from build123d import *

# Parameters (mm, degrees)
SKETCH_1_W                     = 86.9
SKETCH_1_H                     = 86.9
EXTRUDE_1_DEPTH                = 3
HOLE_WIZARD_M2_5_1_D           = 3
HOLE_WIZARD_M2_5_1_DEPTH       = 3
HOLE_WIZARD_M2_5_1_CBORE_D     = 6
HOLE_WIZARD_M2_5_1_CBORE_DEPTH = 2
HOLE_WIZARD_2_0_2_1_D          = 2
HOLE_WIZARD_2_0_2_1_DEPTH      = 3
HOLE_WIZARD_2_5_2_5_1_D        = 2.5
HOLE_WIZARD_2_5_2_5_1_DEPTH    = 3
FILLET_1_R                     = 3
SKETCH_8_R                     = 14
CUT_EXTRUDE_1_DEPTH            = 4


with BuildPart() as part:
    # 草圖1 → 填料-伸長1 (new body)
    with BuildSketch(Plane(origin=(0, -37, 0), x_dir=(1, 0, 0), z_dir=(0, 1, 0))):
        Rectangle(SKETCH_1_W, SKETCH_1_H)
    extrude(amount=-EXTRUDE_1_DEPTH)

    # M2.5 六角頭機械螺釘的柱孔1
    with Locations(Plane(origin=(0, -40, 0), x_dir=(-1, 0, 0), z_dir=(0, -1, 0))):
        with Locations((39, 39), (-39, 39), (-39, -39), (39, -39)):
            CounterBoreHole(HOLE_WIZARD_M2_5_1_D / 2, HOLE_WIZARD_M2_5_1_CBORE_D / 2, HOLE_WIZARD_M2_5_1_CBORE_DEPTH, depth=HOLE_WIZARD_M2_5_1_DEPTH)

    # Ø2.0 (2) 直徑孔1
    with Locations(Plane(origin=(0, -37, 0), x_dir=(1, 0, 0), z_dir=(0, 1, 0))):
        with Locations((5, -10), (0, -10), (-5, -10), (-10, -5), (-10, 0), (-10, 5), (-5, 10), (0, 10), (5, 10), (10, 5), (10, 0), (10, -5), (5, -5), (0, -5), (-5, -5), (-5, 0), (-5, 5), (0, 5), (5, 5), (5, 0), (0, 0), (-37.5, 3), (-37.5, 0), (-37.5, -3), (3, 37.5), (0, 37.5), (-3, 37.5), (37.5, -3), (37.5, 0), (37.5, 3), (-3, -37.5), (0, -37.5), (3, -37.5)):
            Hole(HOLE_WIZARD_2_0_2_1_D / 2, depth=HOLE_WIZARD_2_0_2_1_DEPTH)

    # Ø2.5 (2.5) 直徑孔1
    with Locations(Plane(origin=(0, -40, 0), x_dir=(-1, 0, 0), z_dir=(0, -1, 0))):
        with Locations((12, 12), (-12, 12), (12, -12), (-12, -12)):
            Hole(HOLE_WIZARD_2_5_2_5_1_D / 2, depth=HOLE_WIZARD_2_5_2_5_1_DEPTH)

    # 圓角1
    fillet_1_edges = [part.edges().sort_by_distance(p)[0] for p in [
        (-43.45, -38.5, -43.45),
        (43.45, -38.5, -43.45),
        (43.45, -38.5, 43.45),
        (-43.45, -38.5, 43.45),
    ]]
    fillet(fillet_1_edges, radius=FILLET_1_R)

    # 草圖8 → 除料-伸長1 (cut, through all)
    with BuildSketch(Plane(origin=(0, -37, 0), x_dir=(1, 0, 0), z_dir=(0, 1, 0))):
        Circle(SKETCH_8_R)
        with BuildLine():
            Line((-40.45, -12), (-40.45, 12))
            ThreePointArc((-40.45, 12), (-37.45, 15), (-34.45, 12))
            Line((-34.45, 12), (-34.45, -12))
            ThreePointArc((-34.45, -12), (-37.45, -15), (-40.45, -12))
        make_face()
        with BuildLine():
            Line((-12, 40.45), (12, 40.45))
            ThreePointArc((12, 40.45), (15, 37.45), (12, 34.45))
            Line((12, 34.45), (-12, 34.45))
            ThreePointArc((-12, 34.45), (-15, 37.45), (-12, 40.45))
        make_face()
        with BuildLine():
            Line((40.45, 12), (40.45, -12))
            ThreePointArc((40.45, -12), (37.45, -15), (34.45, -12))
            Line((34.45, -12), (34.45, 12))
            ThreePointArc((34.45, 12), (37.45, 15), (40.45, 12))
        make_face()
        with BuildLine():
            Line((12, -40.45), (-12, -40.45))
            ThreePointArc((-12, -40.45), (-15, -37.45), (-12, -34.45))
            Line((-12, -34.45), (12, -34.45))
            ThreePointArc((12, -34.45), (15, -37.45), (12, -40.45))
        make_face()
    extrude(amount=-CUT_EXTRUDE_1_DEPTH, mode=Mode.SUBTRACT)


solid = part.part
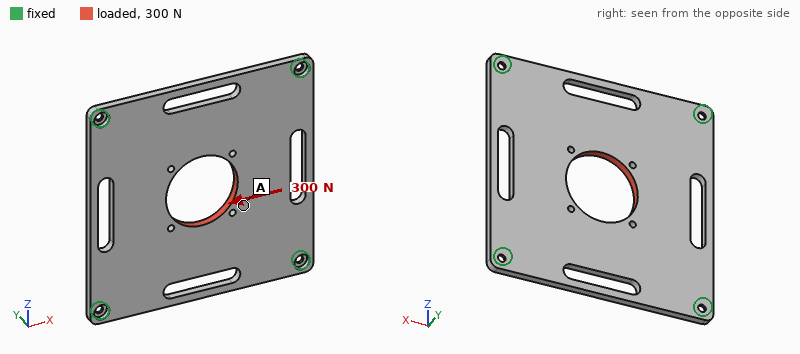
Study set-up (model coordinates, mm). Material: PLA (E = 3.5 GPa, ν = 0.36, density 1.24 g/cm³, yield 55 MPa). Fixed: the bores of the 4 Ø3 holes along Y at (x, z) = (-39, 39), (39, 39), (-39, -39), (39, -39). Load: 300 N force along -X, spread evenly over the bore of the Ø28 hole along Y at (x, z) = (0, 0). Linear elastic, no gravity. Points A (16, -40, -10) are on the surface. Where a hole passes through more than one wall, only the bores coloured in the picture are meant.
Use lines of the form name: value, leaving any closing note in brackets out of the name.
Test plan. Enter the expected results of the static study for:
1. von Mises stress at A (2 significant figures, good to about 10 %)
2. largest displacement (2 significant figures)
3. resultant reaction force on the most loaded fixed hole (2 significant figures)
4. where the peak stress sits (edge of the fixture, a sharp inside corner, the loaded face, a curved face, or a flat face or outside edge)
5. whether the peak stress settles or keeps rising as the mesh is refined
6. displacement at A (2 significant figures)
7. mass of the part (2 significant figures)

von Mises stress at A: 1.2 MPa
largest displacement: 57 µm
resultant reaction force on the most loaded fixed hole: 84 N
where the peak stress sits: edge of the fixture
whether the peak stress settles or keeps rising as the mesh is refined: keeps rising
displacement at A: 43 µm
mass of the part: 23 g
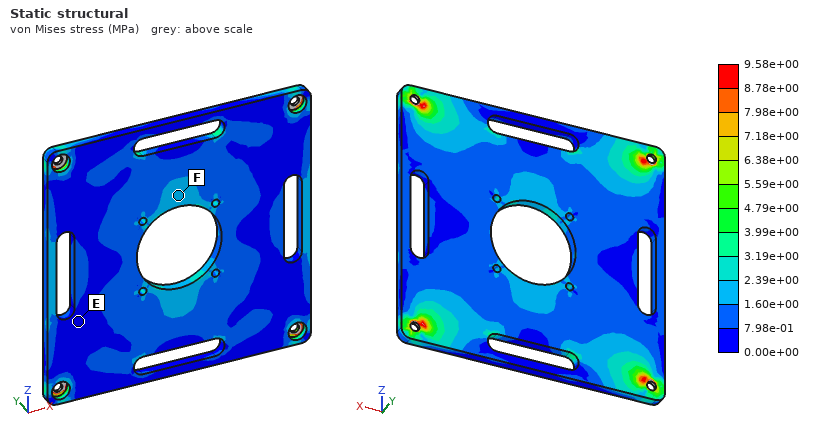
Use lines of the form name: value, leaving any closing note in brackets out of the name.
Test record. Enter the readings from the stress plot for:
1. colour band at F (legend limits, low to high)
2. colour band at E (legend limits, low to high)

colour band at F: 1.60e+00 to 2.39e+00 MPa
colour band at E: 0.00e+00 to 7.98e-01 MPa
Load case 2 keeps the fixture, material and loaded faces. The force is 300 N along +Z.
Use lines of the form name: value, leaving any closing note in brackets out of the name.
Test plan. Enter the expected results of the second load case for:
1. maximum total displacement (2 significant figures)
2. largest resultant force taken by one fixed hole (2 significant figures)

maximum total displacement: 57 µm
largest resultant force taken by one fixed hole: 84 N
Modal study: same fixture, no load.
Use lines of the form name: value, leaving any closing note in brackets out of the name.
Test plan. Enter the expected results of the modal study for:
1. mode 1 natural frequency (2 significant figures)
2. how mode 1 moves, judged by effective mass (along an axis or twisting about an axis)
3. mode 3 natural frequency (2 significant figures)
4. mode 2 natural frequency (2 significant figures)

mode 1 natural frequency: 420 Hz
how mode 1 moves, judged by effective mass: along Y
mode 3 natural frequency: 770 Hz
mode 2 natural frequency: 770 Hz
